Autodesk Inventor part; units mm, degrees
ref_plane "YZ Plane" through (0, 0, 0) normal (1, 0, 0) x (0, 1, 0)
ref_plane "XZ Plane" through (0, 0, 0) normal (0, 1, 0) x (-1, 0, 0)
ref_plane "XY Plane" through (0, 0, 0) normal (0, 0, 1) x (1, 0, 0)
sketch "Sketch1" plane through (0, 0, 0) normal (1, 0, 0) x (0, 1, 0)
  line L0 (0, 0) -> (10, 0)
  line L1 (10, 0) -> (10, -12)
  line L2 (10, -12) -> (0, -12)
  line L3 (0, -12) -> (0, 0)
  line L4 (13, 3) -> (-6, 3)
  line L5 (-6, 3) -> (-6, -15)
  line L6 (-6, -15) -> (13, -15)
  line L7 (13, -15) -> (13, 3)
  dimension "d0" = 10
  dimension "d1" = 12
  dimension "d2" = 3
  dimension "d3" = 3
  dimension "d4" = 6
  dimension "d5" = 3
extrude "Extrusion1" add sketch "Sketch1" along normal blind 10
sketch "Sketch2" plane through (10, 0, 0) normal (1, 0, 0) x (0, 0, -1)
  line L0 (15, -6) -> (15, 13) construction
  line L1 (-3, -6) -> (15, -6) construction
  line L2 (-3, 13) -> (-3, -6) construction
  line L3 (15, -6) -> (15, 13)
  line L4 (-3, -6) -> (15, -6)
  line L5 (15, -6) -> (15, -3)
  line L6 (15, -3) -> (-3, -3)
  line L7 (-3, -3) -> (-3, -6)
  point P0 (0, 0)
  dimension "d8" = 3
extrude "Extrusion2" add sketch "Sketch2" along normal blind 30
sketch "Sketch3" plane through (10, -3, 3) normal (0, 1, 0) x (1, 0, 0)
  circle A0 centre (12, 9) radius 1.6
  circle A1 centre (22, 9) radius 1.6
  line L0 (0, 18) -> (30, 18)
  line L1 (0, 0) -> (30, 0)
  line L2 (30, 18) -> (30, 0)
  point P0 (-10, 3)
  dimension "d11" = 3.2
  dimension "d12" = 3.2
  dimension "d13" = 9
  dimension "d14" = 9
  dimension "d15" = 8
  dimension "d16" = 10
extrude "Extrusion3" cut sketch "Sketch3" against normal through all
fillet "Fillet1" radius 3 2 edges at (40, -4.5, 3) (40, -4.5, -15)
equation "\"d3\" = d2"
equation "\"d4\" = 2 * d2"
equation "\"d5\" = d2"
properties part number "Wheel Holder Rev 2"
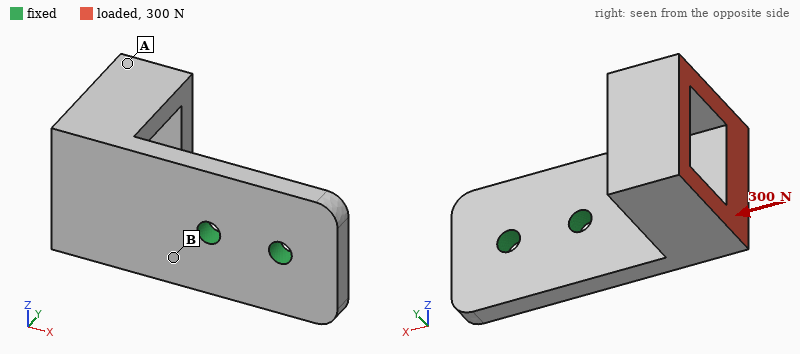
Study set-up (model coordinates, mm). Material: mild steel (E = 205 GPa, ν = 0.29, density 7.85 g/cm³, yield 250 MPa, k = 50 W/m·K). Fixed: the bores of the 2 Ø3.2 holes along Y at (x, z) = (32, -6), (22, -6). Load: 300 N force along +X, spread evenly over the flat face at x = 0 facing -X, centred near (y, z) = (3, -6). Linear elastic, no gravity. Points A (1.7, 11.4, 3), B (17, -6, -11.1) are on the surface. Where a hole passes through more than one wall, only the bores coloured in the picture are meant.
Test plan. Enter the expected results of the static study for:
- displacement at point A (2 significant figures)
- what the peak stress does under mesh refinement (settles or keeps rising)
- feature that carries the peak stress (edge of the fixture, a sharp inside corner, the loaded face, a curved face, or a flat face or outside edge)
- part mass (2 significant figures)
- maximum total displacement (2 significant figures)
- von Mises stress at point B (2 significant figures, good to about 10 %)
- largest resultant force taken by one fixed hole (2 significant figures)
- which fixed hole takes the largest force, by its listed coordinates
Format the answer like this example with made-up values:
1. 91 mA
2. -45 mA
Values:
1. 74 µm
2. keeps rising
3. edge of the fixture
4. 30 g
5. 82 µm
6. 69 MPa
7. 240 N
8. (22, -6)
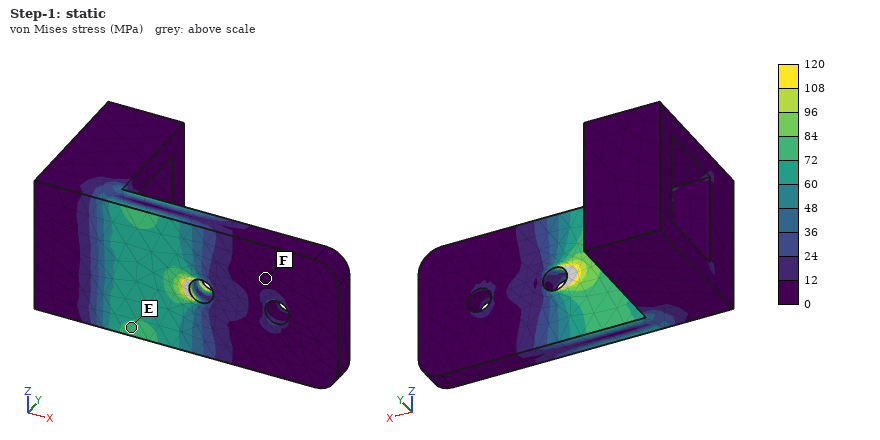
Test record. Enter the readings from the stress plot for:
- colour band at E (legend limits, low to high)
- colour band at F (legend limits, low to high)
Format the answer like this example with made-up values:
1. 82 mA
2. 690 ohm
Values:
1. 72 to 84 MPa
2. 0 to 12 MPa
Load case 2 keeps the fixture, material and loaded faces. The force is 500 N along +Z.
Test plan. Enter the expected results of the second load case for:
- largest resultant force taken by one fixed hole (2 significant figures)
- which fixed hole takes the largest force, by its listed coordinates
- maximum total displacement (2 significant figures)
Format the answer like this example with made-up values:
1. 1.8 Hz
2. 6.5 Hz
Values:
1. 1.2 kN
2. (22, -6)
3. 78 µm
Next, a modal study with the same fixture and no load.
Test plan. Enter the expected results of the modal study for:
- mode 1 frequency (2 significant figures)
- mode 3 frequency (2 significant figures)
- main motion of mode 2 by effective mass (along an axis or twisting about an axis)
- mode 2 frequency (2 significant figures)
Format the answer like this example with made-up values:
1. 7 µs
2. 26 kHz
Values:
1. 2000 Hz
2. 8900 Hz
3. along Z
4. 3400 Hz
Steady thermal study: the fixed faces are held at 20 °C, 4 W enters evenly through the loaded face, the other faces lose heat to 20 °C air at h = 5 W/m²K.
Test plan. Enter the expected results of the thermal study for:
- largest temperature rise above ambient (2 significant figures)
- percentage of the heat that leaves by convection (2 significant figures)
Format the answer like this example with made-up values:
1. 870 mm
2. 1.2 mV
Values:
1. 31 K
2. 5.2 %
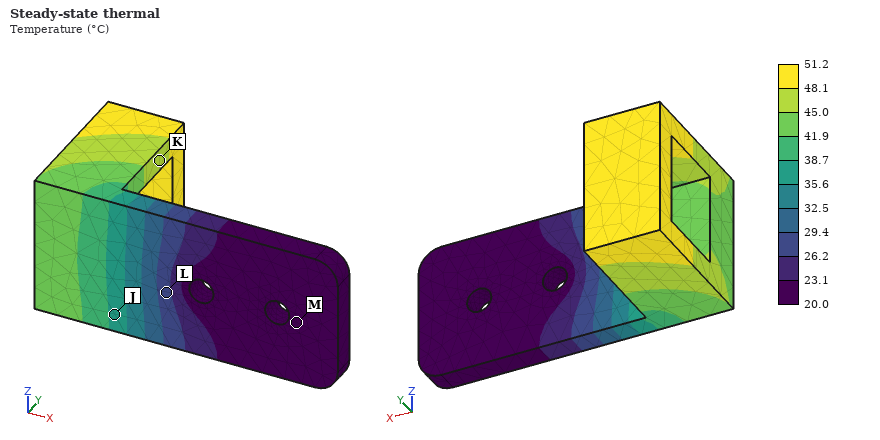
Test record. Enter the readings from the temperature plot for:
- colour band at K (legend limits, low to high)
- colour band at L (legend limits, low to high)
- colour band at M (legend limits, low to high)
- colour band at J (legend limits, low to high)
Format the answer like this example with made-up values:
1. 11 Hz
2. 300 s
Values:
1. 45.0 to 48.1 °C
2. 26.2 to 29.4 °C
3. 20.0 to 23.1 °C
4. 35.6 to 38.7 °C
